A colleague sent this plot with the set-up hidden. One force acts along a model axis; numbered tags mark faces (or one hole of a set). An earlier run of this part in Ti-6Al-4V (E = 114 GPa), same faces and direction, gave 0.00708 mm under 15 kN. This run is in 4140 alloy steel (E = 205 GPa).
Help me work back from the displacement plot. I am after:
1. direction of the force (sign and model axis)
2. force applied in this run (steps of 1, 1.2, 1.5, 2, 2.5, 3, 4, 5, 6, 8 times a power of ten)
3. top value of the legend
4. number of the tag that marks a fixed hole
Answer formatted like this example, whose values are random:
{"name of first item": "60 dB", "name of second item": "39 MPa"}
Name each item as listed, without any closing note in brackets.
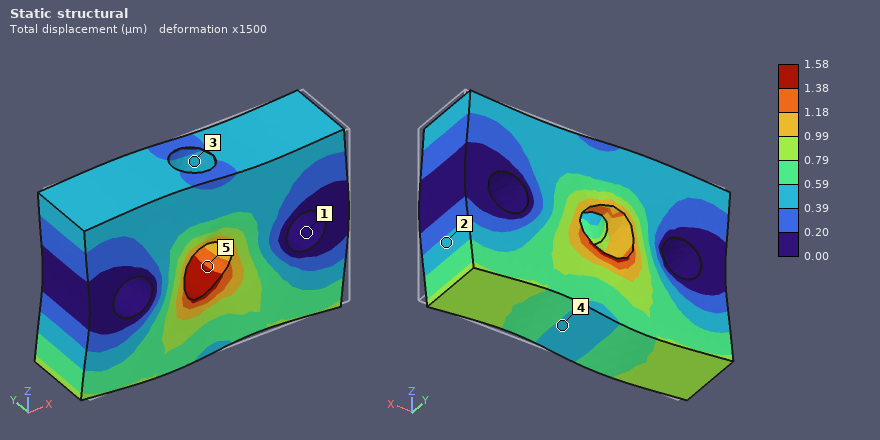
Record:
{"direction of the force": "-X", "force applied in this run": "6 kN", "top value of the legend": "1.58 µm", "number of the tag that marks a fixed hole": "1"}
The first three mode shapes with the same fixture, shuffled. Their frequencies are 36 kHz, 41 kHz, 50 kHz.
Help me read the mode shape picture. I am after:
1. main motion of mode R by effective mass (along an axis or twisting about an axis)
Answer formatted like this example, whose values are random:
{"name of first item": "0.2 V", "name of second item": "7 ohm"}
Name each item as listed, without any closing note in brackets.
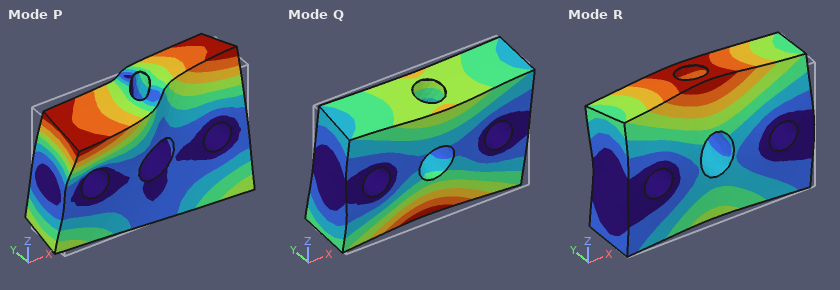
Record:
{"main motion of mode R by effective mass": "along Y"}
